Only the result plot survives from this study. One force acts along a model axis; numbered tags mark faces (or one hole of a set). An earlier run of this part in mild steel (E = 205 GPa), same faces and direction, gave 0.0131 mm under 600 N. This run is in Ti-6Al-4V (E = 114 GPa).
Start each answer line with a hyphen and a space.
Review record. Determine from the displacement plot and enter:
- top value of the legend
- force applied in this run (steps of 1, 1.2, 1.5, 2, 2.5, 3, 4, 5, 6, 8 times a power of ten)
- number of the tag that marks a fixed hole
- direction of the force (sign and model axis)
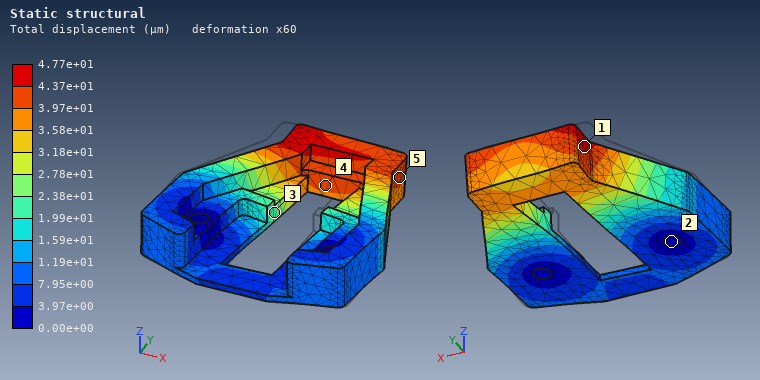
- 4.77e+01 µm
- 1.2 kN
- 2
- +X
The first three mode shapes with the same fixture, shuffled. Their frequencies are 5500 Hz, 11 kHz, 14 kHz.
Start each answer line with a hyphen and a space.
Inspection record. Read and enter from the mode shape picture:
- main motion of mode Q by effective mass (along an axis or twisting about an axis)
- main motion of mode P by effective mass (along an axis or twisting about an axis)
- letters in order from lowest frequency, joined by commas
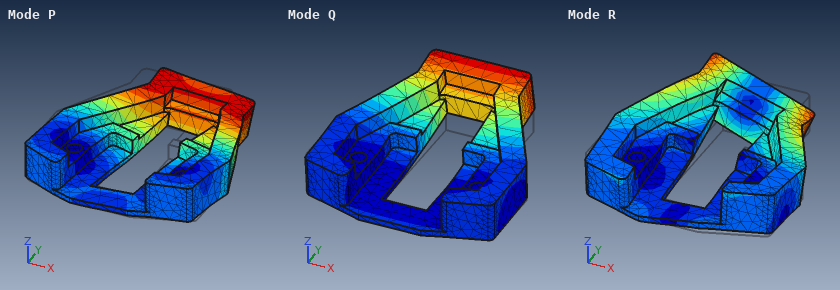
- along Z
- along X
- Q, P, R
